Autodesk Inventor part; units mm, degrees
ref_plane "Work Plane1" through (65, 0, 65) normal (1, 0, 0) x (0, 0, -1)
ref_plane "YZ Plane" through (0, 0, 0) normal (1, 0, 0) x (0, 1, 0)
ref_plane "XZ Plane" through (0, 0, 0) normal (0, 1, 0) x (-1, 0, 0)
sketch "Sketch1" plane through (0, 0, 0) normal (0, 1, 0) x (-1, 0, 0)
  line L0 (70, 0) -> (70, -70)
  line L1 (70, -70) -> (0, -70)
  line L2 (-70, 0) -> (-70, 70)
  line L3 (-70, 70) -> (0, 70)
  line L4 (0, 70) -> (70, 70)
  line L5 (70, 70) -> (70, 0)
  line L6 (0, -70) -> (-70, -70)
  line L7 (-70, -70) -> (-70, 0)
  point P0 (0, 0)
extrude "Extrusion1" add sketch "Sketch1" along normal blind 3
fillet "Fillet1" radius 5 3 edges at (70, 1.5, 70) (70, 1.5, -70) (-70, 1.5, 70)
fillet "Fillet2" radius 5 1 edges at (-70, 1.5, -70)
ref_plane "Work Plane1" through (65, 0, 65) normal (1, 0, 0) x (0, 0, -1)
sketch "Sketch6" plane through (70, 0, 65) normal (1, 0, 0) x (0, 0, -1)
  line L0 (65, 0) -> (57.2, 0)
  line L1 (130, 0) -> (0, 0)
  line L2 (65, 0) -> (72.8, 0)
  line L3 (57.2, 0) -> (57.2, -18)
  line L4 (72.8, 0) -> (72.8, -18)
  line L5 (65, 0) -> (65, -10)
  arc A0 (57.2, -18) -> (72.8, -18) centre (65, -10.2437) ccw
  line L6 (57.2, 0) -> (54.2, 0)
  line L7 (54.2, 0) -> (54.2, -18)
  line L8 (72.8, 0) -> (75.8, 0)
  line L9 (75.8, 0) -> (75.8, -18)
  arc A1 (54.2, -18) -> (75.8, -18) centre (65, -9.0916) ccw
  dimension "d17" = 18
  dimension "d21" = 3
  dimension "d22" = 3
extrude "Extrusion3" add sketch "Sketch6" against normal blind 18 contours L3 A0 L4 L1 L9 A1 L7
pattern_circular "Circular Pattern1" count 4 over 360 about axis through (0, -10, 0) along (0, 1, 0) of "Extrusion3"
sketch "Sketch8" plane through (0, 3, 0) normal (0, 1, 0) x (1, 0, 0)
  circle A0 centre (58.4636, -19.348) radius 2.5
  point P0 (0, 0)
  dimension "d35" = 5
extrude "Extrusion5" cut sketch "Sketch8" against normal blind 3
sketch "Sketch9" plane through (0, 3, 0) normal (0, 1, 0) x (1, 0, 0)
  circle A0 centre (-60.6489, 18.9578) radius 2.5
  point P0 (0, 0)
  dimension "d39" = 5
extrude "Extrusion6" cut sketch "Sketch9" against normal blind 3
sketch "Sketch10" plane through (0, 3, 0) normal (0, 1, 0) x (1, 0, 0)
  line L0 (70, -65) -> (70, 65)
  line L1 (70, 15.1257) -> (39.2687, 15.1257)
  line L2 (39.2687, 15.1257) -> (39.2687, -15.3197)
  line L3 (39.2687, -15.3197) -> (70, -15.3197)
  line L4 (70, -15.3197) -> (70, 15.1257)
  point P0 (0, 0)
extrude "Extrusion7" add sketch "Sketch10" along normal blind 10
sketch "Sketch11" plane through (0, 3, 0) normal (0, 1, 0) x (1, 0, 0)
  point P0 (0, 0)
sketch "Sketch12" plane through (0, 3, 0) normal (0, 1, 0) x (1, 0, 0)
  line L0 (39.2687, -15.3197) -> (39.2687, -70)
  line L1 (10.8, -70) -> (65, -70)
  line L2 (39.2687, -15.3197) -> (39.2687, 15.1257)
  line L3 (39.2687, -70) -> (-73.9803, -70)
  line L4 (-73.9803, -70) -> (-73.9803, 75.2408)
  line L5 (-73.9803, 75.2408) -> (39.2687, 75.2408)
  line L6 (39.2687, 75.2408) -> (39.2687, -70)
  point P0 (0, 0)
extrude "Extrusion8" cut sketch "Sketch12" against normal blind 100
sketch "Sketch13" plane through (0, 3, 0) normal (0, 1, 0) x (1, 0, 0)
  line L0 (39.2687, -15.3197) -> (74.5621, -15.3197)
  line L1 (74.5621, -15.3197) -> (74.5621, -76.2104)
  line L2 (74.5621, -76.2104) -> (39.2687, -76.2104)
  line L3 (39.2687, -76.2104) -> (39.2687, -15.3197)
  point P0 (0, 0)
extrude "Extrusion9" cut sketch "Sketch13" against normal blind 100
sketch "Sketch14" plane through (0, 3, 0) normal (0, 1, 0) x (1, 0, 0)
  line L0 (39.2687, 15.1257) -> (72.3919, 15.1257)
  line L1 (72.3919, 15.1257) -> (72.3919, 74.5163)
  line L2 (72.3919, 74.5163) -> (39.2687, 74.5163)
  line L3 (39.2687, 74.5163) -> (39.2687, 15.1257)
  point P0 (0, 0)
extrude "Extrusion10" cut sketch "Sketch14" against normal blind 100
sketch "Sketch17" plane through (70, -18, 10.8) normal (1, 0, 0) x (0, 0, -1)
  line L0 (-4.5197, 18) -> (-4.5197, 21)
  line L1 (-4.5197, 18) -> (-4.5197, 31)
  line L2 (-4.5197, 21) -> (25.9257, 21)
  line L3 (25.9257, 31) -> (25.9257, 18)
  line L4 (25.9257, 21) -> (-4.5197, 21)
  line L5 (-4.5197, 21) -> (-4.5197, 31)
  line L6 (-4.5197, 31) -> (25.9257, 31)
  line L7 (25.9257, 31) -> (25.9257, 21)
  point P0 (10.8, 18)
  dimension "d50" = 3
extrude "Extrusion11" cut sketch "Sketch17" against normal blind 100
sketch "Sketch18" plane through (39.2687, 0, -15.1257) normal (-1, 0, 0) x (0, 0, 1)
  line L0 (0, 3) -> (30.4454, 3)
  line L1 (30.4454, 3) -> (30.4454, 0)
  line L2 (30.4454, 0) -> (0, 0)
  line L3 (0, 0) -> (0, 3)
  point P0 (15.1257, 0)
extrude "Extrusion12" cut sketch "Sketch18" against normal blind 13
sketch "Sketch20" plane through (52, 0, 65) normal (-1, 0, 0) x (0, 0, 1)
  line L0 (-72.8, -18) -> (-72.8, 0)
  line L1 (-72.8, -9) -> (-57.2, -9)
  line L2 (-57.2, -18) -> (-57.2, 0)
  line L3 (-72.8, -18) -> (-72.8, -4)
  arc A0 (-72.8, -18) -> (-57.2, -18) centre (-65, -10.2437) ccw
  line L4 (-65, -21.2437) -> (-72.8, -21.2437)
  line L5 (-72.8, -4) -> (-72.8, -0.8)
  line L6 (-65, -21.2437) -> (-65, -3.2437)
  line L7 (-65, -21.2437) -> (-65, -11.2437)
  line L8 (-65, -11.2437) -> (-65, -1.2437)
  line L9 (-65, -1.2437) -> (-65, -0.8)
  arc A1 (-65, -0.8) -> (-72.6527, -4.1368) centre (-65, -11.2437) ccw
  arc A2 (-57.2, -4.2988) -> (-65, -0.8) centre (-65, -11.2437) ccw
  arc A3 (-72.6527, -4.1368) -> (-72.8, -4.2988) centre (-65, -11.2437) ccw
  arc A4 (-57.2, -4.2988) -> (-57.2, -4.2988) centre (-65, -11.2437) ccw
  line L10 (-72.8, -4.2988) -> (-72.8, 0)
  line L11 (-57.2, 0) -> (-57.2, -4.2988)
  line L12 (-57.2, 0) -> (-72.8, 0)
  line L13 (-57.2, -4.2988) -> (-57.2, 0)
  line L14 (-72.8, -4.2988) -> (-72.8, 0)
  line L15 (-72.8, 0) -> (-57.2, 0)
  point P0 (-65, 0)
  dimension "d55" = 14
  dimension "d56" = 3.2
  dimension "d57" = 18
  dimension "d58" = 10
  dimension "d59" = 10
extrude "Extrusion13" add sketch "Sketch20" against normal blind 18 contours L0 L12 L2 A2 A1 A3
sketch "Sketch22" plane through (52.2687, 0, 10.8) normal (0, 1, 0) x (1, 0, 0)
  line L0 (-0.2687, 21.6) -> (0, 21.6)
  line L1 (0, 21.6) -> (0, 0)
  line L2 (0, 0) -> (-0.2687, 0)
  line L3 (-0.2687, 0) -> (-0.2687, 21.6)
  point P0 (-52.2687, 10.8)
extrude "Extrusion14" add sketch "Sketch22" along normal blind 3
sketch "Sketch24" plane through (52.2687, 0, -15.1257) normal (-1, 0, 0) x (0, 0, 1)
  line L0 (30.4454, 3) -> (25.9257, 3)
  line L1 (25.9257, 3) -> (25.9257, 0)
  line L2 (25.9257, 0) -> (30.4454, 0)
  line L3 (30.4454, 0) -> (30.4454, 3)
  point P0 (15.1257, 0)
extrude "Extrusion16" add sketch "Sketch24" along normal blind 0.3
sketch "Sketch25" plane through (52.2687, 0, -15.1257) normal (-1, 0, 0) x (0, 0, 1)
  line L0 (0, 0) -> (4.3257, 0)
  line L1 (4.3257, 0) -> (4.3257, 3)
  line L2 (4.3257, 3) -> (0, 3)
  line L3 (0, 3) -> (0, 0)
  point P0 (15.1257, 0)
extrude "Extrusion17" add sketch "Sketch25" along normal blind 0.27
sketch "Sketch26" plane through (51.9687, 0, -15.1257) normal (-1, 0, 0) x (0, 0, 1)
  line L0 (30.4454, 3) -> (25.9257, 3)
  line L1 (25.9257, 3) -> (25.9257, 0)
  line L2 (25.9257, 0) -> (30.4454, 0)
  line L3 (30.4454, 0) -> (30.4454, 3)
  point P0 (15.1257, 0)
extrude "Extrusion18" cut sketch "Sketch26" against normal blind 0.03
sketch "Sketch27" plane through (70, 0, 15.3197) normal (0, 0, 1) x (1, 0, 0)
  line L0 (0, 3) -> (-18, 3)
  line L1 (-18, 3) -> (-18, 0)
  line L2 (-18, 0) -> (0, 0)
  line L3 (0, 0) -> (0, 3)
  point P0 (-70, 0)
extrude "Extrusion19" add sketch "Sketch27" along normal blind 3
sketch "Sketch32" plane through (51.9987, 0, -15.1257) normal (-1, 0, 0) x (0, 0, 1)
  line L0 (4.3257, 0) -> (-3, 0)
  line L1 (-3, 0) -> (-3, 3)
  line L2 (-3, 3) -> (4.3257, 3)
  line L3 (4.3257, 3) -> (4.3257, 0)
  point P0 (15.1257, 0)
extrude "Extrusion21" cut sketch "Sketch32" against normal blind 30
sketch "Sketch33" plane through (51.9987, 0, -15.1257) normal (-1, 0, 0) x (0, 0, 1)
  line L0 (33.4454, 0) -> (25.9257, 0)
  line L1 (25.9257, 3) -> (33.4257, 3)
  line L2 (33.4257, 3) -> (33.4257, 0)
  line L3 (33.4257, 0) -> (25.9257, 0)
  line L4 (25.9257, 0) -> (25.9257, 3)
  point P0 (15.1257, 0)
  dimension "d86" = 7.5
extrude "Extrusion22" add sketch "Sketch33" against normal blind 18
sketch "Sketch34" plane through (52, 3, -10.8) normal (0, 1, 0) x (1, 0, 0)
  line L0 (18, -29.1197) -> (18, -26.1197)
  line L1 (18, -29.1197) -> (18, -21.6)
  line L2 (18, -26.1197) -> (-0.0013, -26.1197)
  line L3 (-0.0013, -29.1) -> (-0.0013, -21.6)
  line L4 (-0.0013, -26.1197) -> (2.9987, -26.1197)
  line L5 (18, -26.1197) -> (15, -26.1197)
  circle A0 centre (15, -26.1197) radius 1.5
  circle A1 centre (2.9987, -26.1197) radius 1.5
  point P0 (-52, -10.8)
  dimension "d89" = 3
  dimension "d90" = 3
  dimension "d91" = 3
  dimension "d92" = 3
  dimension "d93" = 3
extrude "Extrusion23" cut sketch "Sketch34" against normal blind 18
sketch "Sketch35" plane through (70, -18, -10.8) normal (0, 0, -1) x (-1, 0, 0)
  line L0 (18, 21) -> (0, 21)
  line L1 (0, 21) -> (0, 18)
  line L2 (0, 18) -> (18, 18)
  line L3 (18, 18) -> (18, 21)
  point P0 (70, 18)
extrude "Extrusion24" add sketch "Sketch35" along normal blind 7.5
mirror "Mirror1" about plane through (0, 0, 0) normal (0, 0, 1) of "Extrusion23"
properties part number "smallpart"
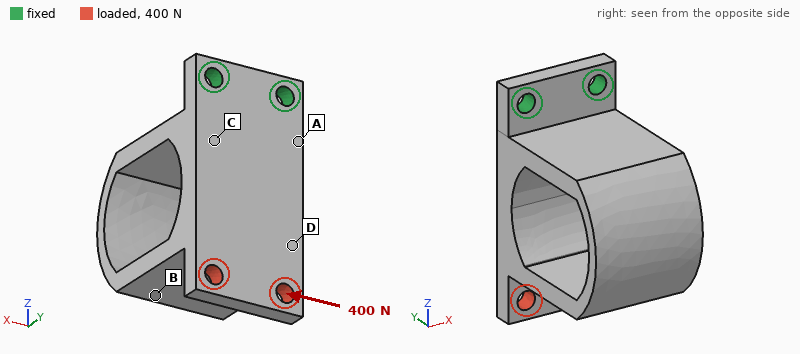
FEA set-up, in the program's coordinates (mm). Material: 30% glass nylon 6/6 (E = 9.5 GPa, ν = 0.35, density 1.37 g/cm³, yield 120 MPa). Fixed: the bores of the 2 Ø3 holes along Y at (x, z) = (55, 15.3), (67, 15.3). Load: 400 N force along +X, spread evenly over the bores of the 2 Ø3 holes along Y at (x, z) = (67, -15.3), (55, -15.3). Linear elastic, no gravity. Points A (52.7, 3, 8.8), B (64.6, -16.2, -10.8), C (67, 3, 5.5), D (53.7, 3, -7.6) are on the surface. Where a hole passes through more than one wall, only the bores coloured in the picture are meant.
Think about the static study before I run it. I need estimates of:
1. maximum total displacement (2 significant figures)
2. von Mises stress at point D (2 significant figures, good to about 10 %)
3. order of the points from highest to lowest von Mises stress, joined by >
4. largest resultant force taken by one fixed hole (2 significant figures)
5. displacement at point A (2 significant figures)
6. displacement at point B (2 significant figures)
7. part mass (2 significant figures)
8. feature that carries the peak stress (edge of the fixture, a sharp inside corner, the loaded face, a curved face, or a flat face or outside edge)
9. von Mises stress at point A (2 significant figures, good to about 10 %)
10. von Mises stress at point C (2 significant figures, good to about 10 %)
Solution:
0.35 mm
15 MPa
A > C > D > B
940 N
0.052 mm
0.15 mm
7.0 g
a flat face or outside edge
51 MPa
33 MPa
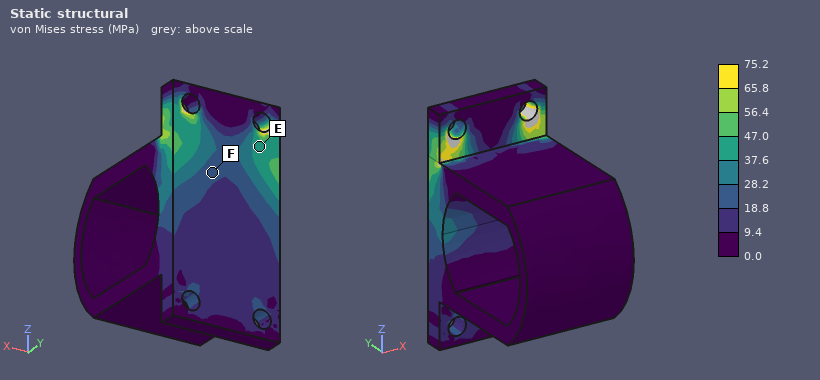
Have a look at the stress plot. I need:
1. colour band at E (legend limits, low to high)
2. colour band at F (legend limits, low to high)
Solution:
37.6 to 47.0 MPa
18.8 to 28.2 MPa
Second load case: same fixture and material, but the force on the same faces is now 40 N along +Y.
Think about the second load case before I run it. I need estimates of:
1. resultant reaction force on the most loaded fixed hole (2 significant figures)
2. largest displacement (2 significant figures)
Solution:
20 N
0.57 mm
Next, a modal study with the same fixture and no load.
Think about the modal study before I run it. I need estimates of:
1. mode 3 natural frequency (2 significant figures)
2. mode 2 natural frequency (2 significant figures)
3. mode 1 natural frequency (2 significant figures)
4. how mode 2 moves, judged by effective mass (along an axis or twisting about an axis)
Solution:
4300 Hz
2600 Hz
810 Hz
along X
